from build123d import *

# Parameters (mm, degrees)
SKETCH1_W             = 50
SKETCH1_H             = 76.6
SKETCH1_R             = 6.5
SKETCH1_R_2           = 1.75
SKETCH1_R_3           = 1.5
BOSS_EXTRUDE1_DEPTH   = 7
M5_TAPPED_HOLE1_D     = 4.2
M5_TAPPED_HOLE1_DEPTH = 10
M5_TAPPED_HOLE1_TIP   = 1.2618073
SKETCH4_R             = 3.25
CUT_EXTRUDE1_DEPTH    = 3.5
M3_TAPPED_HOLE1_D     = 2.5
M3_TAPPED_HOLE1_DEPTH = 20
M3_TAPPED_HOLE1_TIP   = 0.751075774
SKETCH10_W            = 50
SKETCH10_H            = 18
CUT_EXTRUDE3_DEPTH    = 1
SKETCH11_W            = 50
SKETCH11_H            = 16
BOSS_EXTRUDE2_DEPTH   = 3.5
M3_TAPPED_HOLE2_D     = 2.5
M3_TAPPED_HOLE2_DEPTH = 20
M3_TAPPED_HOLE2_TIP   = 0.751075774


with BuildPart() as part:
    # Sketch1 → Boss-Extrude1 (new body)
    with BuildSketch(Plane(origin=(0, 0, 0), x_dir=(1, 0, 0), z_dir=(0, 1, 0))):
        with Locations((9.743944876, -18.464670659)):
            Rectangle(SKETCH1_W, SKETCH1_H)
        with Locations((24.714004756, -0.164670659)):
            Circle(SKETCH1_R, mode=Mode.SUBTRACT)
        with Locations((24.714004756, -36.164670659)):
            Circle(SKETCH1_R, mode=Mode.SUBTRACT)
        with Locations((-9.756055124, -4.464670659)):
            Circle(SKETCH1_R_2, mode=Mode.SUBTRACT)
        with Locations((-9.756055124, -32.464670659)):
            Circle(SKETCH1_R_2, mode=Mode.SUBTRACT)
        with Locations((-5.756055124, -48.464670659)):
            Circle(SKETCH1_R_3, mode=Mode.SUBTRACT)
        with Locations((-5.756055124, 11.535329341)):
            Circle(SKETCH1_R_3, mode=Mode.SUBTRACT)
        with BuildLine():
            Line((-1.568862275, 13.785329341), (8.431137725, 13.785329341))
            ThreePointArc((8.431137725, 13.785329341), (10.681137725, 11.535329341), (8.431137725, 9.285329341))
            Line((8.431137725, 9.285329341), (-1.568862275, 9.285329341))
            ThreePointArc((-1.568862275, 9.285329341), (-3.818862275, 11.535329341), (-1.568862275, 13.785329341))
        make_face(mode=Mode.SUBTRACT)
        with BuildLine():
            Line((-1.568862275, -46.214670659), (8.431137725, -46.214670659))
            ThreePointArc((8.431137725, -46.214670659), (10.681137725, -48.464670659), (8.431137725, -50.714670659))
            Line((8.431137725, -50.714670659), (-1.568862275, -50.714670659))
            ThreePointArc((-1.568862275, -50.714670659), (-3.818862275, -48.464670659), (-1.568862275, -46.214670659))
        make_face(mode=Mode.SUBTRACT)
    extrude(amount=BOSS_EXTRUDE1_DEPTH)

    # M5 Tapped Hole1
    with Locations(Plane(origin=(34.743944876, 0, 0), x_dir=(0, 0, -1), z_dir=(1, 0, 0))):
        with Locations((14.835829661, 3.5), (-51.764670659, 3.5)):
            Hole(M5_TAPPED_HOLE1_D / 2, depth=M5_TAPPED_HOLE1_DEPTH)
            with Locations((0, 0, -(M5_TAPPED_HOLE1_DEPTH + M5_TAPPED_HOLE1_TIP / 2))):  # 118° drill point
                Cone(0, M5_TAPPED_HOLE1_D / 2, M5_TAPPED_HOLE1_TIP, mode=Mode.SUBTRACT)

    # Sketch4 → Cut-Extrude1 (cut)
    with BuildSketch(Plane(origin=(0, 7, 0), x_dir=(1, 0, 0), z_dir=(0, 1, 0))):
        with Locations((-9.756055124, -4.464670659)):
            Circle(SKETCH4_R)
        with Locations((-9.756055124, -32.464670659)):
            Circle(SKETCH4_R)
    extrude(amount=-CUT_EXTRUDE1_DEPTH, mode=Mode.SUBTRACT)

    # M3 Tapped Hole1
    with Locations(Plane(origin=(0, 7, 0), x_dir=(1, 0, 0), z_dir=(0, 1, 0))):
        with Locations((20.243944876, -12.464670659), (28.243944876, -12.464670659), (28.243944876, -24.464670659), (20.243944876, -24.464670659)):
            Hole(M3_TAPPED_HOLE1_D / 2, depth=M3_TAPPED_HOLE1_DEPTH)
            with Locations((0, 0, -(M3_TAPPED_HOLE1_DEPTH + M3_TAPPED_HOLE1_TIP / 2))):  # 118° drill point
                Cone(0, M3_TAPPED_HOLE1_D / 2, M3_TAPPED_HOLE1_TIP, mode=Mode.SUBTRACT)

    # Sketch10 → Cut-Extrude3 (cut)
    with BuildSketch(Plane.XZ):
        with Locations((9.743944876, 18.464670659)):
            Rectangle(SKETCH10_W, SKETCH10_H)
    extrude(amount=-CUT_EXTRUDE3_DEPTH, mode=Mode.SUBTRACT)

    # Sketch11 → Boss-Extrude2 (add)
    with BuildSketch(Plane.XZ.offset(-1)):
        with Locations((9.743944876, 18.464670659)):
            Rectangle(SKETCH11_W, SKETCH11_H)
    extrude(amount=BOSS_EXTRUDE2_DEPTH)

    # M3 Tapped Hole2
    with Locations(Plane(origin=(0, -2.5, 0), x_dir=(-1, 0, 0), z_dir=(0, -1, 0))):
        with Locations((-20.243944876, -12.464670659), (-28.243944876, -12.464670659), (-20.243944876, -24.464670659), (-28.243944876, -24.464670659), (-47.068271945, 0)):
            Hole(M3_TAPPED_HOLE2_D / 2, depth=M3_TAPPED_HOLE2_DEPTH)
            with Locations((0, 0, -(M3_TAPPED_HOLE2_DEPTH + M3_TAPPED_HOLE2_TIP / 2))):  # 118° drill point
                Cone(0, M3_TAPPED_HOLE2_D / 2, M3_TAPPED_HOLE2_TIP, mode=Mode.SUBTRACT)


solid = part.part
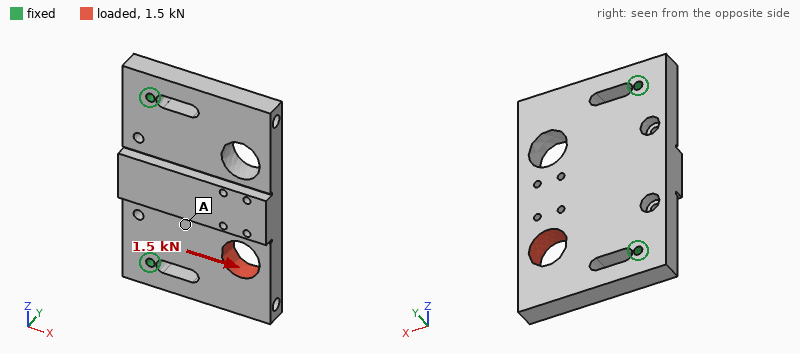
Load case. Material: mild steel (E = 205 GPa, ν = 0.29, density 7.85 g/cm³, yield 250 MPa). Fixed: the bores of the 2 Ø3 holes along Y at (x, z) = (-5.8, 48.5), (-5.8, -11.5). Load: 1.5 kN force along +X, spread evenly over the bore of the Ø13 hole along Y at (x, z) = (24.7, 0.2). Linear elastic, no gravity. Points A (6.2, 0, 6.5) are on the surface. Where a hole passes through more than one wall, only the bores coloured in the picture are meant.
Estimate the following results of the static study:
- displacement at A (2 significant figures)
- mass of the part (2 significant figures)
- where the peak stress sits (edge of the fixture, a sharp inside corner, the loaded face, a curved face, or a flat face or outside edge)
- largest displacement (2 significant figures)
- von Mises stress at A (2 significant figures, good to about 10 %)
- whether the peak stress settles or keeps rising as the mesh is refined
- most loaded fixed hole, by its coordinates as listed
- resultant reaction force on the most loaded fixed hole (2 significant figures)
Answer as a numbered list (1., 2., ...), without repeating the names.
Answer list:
1. 1.4 µm
2. 200 g
3. edge of the fixture
4. 3.1 µm
5. 4.1 MPa
6. keeps rising
7. (-5.8, -11.5)
8. 1.2 kN
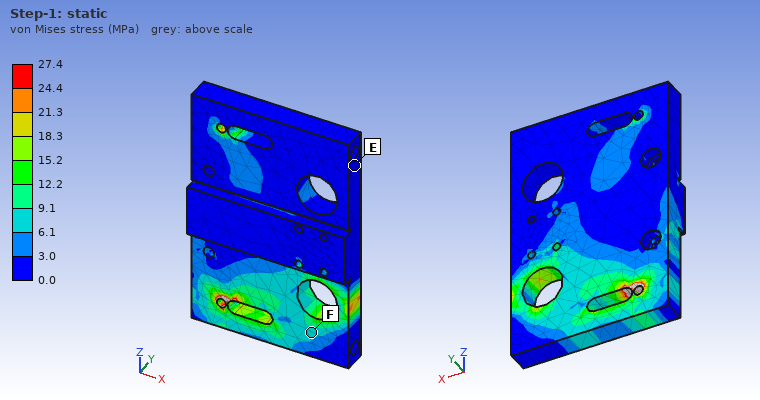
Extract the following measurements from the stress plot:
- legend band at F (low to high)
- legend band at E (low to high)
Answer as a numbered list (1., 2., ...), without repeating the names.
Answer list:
1. 6.1 to 9.1 MPa
2. 0.0 to 3.0 MPa
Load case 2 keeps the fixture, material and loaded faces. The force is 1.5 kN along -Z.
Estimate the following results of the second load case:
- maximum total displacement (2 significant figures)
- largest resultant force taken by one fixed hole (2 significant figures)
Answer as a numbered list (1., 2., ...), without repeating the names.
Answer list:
1. 4.5 µm
2. 1.1 kN
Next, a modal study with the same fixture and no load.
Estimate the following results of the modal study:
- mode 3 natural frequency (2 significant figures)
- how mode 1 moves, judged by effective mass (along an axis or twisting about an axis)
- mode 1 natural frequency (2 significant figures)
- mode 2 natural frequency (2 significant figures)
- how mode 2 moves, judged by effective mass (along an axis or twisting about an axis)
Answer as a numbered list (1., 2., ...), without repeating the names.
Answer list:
1. 7100 Hz
2. along Y
3. 2200 Hz
4. 4900 Hz
5. twisting about X
